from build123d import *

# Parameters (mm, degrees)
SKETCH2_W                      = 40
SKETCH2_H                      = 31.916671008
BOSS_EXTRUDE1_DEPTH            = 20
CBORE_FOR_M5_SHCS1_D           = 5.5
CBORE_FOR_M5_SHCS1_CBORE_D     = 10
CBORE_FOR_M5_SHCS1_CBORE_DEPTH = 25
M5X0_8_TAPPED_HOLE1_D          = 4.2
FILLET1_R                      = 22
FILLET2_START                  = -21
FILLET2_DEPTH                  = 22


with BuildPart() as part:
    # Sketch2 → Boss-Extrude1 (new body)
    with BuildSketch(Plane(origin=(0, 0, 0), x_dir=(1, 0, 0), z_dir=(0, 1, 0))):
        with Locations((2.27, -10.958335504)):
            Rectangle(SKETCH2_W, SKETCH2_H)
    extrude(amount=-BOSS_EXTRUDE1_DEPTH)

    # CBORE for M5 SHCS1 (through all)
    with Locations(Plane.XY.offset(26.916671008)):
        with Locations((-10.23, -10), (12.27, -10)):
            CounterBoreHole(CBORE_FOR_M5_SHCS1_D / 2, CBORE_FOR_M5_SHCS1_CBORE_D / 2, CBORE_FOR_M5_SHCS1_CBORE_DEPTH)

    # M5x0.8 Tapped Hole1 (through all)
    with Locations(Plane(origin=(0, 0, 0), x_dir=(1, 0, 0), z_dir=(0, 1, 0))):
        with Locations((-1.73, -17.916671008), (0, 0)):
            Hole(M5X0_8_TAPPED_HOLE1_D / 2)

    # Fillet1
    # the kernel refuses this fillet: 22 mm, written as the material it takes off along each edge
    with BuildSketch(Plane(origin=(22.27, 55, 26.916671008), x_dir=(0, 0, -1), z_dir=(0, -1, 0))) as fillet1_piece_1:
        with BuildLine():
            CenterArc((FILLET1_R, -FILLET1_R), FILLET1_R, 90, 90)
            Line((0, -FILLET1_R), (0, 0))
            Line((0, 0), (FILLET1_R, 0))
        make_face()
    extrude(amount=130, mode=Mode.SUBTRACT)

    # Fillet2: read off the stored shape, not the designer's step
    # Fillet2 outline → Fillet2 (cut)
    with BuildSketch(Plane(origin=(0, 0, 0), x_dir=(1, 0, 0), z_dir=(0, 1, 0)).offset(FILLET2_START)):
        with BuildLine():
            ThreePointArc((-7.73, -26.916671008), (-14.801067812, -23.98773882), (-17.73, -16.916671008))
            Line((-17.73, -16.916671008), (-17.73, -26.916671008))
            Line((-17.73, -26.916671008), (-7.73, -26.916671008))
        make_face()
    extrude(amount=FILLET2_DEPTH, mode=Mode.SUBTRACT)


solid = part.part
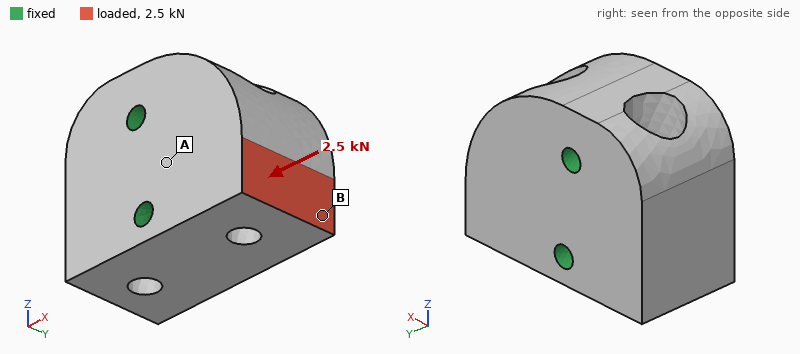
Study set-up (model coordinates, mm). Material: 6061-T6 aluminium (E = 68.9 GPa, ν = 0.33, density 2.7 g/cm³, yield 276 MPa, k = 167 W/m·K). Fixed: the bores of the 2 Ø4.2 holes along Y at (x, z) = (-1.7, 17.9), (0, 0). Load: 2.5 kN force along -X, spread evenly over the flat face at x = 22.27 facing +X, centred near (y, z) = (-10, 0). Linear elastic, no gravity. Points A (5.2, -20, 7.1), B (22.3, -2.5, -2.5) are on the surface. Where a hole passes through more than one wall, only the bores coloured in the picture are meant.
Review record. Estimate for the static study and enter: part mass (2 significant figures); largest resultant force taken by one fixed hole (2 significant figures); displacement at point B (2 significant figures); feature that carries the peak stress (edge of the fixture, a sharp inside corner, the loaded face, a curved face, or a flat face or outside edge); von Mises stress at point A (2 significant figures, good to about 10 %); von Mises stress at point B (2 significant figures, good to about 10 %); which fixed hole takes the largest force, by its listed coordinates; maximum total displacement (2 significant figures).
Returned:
50 g
2.4 kN
5.6 µm
a curved face
5.1 MPa
12 MPa
(0, 0)
6.9 µm
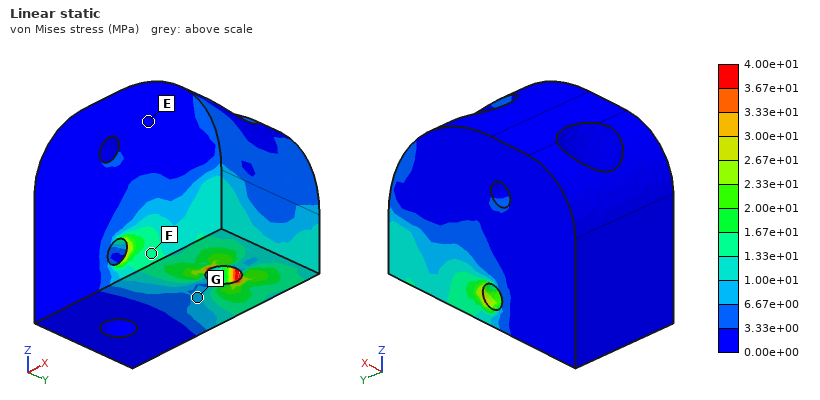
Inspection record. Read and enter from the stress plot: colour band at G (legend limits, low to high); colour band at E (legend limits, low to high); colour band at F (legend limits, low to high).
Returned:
6.67e+00 to 1.00e+01 MPa
0.00e+00 to 3.33e+00 MPa
1.33e+01 to 1.67e+01 MPa
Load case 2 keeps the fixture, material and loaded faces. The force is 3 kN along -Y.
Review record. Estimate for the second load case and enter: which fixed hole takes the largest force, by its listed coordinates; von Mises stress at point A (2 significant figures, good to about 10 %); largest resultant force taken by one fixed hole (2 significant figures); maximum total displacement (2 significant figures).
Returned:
(0, 0)
32 MPa
2.5 kN
33 µm
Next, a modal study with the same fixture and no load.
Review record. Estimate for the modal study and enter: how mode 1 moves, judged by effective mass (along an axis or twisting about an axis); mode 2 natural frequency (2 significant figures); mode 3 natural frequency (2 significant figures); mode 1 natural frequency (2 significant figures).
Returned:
along Y
27 kHz
27 kHz
21 kHz
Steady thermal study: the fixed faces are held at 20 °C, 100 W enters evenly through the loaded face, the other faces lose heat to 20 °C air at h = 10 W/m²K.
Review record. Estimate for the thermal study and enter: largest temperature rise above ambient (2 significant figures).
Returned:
50 K
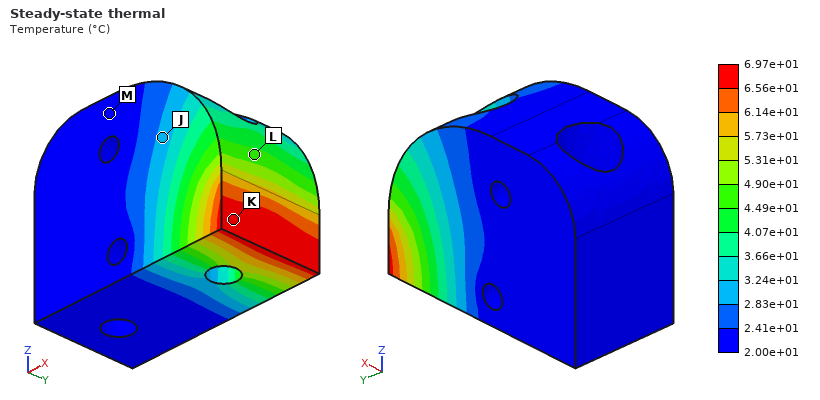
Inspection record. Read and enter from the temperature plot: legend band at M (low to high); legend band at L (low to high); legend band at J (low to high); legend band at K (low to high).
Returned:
2.00e+01 to 2.41e+01 °C
4.49e+01 to 4.90e+01 °C
2.83e+01 to 3.24e+01 °C
6.56e+01 to 6.97e+01 °C
